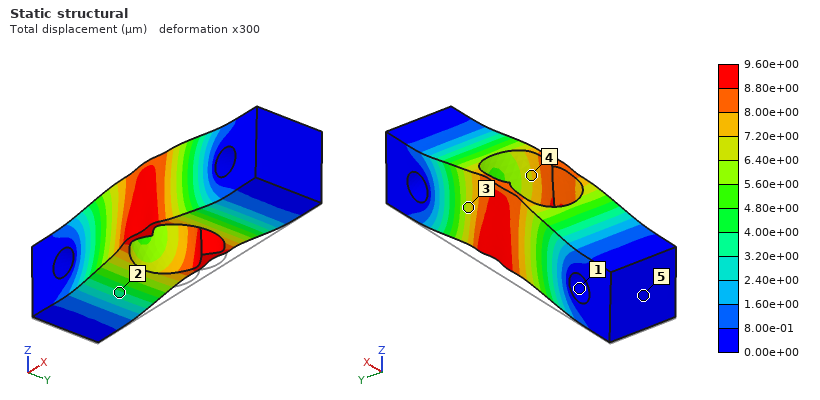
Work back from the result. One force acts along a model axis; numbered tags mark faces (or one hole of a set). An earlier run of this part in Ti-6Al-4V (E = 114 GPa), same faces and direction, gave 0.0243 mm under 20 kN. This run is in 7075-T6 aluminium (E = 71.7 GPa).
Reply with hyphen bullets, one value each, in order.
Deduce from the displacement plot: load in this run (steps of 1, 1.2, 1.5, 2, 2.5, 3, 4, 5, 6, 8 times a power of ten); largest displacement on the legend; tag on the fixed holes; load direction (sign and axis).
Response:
- 5 kN
- 9.60e+00 µm
- 1
- +Z
